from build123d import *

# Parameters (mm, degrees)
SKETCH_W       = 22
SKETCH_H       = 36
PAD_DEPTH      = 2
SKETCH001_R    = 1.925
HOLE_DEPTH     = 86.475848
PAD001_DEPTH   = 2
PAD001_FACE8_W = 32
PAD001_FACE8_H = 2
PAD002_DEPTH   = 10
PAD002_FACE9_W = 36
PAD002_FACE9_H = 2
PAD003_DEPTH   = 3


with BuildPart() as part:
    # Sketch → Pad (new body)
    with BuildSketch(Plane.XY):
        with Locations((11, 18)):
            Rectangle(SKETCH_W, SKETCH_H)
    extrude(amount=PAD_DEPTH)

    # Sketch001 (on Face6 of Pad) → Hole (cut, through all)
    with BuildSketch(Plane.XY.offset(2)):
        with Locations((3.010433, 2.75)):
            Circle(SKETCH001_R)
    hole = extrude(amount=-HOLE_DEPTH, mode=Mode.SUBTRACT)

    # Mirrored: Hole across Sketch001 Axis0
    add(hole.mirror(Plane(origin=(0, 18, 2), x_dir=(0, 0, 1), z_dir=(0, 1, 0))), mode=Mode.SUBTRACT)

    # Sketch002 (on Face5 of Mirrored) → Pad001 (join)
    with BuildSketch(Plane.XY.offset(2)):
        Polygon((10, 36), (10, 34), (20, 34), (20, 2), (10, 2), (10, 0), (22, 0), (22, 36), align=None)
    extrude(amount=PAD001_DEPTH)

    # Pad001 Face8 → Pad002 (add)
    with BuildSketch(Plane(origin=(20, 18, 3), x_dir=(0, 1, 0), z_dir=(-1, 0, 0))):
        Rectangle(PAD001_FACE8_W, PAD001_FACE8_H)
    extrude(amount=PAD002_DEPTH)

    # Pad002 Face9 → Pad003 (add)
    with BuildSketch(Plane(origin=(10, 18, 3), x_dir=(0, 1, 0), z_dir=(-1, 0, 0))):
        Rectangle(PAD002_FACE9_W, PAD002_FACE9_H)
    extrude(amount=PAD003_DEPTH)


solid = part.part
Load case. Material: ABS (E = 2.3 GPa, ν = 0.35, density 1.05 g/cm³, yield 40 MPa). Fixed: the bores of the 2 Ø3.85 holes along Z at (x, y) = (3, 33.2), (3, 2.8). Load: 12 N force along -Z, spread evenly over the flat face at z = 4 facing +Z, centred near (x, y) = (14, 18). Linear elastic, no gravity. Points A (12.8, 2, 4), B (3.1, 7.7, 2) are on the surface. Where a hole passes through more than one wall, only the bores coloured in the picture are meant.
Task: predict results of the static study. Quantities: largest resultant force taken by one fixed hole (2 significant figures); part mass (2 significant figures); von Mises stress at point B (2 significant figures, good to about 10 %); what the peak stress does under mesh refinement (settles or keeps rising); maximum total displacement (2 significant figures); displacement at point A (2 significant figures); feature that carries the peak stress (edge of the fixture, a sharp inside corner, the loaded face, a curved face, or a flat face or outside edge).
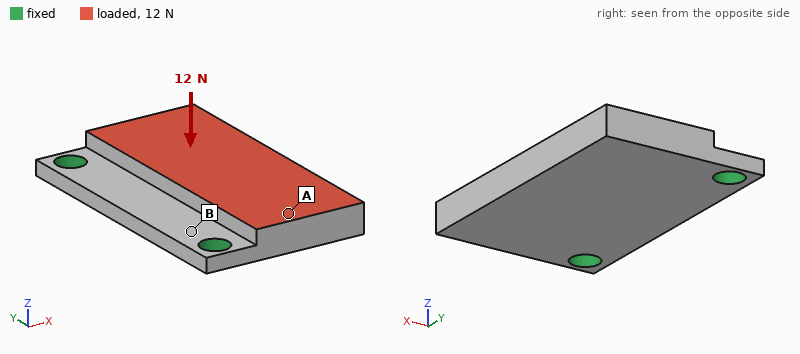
6.3 N
2.7 g
3.2 MPa
keeps rising
0.21 mm
0.088 mm
edge of the fixture
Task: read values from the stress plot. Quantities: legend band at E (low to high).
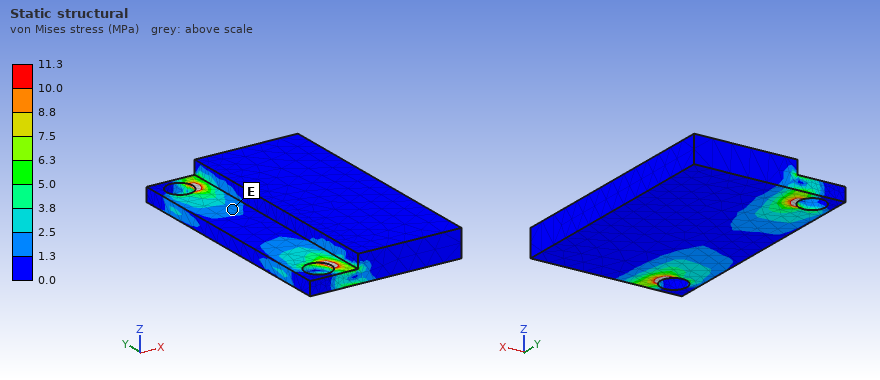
1.3 to 2.5 MPa
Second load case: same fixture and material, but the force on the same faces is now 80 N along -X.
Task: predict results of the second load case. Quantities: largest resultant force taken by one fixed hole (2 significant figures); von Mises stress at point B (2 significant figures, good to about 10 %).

41 N
7.8 MPa
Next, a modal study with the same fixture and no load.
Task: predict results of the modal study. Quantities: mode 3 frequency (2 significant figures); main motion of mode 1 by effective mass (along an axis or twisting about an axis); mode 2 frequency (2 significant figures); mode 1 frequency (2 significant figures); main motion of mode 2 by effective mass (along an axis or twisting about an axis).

4500 Hz
along Z
3000 Hz
980 Hz
twisting about X
